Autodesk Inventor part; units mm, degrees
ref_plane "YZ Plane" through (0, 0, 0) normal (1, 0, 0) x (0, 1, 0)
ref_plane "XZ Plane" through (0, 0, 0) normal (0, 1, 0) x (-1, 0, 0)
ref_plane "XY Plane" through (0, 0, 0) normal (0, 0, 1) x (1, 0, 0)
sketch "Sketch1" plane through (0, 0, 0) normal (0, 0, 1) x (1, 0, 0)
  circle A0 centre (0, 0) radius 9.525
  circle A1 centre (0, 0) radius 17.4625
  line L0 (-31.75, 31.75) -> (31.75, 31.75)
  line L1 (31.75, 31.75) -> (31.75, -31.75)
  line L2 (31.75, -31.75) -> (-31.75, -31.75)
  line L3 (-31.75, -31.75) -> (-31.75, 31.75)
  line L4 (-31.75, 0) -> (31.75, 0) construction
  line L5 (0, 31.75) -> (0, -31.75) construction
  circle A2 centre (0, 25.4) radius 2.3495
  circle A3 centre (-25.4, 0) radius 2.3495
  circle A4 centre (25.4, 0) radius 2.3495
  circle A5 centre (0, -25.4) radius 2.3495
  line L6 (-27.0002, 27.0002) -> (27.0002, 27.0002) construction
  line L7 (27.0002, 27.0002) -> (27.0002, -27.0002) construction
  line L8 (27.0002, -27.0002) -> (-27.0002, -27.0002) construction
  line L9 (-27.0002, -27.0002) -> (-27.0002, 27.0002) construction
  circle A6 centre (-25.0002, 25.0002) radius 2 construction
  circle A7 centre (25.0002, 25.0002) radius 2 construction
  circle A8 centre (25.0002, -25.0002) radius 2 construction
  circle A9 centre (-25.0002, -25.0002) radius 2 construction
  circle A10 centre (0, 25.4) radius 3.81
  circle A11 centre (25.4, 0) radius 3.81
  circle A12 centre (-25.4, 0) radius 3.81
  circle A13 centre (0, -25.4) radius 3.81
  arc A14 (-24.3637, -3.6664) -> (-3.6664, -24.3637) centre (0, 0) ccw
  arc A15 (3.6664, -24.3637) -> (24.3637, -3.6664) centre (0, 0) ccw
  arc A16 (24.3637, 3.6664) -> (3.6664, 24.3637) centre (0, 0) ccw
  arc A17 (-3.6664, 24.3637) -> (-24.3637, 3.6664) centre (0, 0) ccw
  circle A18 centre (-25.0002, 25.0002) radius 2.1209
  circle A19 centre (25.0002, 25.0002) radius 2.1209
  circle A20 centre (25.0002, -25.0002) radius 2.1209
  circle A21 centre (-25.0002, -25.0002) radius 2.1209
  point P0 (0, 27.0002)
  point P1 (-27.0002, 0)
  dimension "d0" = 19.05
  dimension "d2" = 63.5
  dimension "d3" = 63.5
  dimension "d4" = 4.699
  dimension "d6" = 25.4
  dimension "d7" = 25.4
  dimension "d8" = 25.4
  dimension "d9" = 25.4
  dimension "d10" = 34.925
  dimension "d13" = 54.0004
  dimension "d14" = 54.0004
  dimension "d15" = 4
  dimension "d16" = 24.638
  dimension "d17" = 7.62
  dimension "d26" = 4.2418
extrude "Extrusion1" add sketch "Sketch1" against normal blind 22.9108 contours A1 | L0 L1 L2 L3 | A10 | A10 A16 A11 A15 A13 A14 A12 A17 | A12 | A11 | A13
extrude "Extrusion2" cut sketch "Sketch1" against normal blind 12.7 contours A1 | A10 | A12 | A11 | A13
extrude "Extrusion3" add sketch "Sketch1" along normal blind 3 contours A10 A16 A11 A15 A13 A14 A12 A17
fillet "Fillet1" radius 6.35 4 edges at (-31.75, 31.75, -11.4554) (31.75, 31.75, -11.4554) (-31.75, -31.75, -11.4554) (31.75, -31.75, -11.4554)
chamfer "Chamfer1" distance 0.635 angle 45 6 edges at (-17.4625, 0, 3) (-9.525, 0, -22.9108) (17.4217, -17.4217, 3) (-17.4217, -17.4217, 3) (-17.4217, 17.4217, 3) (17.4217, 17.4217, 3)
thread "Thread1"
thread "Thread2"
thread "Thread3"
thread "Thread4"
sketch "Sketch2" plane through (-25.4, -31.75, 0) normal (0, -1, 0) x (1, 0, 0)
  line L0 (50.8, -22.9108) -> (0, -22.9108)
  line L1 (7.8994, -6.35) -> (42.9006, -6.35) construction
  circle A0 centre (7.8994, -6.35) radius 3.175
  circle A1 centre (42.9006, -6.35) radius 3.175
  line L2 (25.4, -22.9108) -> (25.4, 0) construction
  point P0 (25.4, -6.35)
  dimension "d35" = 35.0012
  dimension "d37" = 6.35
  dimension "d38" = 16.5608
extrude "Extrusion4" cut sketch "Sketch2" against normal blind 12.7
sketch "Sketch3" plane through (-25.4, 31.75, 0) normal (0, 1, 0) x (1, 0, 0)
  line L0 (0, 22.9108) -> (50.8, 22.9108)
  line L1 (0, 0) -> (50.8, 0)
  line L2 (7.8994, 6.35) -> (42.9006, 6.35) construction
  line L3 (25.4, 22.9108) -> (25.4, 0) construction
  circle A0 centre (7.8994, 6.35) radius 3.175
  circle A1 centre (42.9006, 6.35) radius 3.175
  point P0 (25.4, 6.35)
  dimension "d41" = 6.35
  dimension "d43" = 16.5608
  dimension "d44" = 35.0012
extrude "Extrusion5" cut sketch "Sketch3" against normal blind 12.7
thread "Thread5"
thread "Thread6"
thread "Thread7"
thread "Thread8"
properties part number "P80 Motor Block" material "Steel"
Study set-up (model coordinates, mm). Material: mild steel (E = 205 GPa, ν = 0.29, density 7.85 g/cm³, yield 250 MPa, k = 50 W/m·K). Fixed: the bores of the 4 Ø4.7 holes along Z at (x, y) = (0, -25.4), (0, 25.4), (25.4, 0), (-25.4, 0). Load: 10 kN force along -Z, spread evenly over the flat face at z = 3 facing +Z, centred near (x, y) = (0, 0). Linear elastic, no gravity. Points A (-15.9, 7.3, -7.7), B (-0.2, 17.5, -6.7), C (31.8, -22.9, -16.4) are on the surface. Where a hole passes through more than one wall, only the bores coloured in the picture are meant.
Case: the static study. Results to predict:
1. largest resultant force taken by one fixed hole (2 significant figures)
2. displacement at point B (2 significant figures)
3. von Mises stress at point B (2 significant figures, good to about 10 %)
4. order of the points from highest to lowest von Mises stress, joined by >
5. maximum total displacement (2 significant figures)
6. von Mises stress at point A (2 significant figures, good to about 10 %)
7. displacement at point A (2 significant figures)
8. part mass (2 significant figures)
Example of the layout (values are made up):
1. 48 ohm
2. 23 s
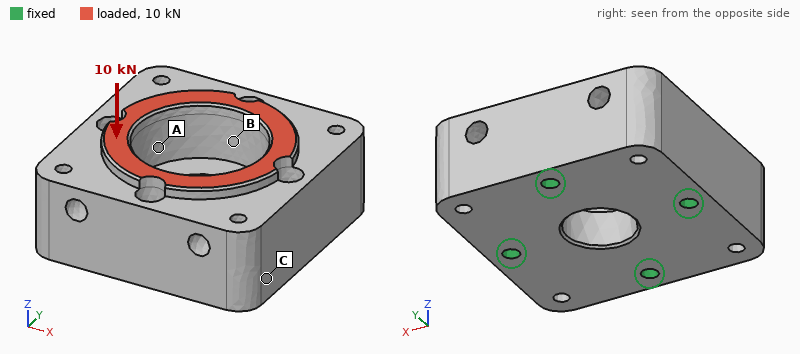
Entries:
1. 2.6 kN
2. 1.1 µm
3. 13 MPa
4. B > A > C
5. 1.7 µm
6. 9.6 MPa
7. 1.2 µm
8. 570 g
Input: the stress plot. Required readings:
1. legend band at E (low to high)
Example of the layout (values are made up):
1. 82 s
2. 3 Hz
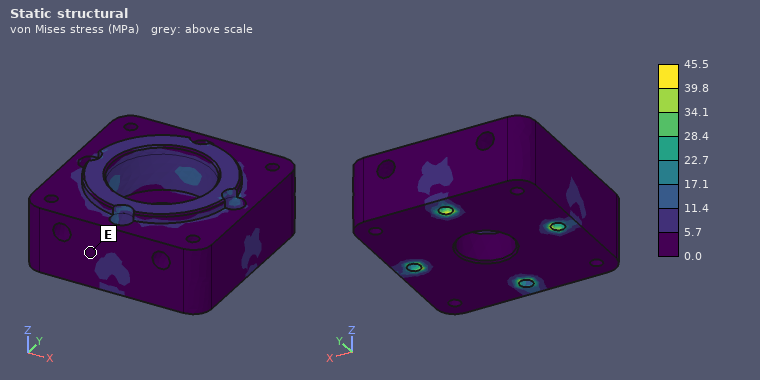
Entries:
1. 0.0 to 5.7 MPa
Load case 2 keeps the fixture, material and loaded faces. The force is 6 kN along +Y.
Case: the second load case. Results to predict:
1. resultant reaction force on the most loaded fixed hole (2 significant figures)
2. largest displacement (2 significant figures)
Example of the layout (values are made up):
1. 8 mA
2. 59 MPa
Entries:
1. 2.4 kN
2. 4.1 µm
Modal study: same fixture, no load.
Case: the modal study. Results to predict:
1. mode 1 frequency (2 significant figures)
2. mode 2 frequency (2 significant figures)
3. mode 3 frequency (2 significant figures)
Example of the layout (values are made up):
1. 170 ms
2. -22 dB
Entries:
1. 13 kHz
2. 15 kHz
3. 15 kHz
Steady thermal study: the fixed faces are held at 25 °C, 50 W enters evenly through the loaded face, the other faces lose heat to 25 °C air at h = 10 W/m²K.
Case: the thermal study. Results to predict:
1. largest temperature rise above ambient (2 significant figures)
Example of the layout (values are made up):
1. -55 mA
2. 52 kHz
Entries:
1. 19 K
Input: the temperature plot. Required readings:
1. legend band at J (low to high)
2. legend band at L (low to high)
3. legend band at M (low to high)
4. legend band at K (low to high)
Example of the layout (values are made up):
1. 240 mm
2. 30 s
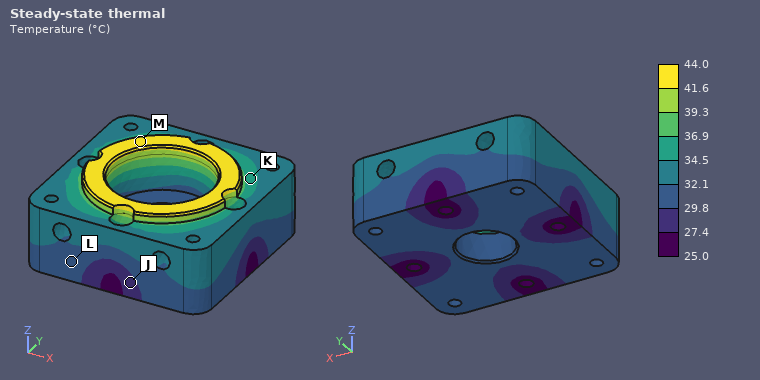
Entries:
1. 27.4 to 29.8 °C
2. 29.8 to 32.1 °C
3. 41.6 to 44.0 °C
4. 34.5 to 36.9 °C
